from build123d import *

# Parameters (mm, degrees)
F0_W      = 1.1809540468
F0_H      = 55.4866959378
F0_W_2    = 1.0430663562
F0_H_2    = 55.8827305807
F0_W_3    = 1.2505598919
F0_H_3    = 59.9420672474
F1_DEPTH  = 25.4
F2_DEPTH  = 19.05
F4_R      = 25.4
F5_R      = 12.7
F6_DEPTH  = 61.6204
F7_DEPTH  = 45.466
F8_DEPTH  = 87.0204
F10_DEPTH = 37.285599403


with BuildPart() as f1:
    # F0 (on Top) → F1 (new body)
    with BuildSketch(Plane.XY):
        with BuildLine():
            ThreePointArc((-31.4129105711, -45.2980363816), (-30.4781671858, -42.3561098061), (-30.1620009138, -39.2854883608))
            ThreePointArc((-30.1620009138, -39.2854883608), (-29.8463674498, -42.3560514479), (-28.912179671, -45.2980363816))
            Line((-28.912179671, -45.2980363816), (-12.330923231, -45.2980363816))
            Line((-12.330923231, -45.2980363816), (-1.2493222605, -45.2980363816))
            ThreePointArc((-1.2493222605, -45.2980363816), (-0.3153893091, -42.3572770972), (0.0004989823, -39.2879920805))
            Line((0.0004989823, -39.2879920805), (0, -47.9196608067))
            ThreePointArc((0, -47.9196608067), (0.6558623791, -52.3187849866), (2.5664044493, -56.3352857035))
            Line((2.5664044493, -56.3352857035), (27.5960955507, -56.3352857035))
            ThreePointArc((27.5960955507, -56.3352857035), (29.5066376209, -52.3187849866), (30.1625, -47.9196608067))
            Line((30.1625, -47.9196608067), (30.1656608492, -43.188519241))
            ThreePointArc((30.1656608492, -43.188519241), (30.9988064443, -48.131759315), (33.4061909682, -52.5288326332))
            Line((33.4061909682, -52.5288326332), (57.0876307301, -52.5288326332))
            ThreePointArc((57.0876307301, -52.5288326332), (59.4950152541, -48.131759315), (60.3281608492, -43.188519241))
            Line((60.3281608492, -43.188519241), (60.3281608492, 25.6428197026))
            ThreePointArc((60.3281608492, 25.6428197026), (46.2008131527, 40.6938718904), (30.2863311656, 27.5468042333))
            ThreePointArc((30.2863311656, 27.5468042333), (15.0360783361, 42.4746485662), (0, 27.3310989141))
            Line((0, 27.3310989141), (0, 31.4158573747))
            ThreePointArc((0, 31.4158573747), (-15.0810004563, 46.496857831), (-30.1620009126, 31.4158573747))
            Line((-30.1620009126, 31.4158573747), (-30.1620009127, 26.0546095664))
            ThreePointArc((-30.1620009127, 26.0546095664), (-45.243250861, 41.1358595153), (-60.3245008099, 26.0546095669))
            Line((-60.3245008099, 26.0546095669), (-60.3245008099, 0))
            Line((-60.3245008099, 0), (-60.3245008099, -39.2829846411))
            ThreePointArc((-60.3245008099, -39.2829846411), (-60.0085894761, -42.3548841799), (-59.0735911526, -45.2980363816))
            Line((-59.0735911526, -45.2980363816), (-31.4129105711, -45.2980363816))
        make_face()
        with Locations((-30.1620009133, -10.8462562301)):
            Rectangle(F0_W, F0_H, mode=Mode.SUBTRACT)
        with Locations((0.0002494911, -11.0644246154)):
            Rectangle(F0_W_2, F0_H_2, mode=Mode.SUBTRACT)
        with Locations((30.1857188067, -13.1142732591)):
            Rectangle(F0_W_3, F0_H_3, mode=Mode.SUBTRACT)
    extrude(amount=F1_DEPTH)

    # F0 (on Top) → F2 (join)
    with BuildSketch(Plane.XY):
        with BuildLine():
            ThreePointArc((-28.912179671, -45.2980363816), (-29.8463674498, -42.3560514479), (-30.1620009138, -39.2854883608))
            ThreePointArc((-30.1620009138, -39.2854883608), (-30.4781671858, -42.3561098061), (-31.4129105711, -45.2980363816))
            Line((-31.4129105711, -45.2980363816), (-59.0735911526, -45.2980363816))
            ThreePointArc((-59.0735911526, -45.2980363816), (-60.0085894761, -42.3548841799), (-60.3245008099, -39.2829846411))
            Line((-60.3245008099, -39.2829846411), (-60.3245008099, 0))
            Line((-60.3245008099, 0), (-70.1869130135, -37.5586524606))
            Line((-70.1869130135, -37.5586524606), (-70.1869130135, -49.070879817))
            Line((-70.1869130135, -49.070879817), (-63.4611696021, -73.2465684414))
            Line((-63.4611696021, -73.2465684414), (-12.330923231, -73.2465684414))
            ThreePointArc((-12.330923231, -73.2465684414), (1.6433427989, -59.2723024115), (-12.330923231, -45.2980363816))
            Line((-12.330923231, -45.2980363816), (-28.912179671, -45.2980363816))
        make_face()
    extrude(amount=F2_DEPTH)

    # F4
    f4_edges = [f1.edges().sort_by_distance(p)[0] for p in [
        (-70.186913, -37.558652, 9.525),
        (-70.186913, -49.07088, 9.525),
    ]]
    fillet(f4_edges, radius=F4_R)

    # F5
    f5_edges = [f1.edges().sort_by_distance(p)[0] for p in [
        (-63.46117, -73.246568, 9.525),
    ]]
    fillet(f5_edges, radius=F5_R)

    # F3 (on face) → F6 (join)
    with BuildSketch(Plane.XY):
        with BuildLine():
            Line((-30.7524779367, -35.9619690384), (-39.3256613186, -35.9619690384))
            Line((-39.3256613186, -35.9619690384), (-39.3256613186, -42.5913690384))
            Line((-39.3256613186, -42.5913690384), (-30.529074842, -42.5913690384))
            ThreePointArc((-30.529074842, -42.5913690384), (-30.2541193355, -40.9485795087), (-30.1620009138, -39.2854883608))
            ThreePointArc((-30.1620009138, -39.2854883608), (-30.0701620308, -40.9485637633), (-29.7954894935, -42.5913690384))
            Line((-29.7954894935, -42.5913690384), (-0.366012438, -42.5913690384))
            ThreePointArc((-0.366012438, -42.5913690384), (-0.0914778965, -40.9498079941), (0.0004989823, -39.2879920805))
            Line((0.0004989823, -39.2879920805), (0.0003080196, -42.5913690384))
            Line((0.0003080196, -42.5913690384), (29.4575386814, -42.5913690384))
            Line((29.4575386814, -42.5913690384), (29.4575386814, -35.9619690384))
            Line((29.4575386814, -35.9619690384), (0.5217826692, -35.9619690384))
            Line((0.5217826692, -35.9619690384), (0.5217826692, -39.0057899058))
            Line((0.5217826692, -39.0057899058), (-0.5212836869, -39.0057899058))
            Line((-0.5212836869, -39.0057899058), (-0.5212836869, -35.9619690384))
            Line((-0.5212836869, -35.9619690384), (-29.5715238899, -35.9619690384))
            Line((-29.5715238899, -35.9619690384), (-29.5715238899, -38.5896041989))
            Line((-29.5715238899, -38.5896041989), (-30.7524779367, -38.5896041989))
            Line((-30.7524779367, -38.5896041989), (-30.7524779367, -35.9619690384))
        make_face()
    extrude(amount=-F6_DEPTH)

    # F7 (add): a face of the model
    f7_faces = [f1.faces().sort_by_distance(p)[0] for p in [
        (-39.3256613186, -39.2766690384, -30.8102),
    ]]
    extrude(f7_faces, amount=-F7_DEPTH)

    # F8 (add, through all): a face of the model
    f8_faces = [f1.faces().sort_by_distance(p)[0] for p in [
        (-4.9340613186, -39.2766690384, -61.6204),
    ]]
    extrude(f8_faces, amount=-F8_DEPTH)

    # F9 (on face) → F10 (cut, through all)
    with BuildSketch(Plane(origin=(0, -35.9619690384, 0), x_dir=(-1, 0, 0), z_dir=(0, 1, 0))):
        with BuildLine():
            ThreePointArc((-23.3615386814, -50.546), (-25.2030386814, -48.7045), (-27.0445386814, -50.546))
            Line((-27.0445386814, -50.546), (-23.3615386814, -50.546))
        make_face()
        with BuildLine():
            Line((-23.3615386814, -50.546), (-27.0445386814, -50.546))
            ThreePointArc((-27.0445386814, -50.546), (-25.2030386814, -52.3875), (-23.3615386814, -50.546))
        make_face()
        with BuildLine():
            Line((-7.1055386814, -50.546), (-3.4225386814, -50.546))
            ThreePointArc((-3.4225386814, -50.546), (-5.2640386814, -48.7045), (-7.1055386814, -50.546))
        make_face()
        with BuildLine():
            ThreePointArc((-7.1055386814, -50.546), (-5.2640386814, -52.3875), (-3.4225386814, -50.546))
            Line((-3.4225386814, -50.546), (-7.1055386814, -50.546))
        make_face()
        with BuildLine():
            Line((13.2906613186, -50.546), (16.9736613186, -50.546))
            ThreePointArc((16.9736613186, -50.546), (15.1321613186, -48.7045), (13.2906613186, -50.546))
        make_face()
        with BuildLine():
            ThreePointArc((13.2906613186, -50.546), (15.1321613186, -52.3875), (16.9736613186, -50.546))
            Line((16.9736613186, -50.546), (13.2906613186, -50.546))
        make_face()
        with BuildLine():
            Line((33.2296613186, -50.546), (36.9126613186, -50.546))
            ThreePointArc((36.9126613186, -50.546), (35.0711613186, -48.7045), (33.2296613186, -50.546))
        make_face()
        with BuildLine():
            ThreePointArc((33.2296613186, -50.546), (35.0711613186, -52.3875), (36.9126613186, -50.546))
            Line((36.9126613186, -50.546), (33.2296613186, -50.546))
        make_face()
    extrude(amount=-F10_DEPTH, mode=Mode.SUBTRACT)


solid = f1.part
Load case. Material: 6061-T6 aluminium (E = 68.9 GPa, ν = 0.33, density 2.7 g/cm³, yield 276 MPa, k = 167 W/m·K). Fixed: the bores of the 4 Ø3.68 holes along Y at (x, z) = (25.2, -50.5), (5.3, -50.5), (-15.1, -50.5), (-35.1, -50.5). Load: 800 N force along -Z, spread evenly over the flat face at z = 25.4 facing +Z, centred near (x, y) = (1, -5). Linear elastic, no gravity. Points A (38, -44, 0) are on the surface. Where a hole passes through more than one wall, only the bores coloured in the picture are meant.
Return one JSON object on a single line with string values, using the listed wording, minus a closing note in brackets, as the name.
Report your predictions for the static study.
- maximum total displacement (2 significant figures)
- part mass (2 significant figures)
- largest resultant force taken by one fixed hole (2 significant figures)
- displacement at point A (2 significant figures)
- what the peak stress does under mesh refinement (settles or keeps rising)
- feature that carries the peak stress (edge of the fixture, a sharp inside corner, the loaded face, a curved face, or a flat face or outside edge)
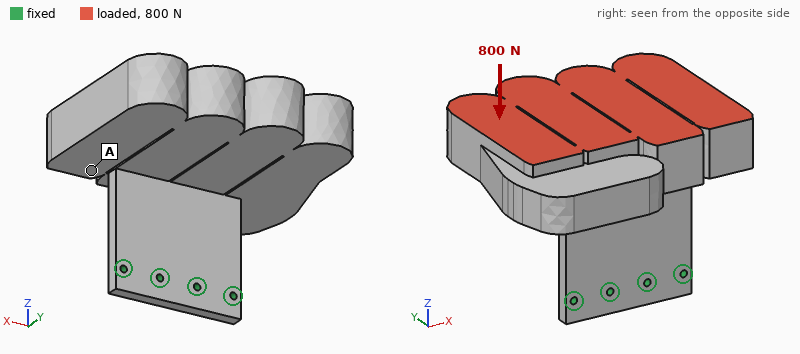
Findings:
{"maximum total displacement": "1.2 mm", "part mass": "910 g", "largest resultant force taken by one fixed hole": "280 N", "displacement at point A": "0.30 mm", "what the peak stress does under mesh refinement": "keeps rising", "feature that carries the peak stress": "edge of the fixture"}
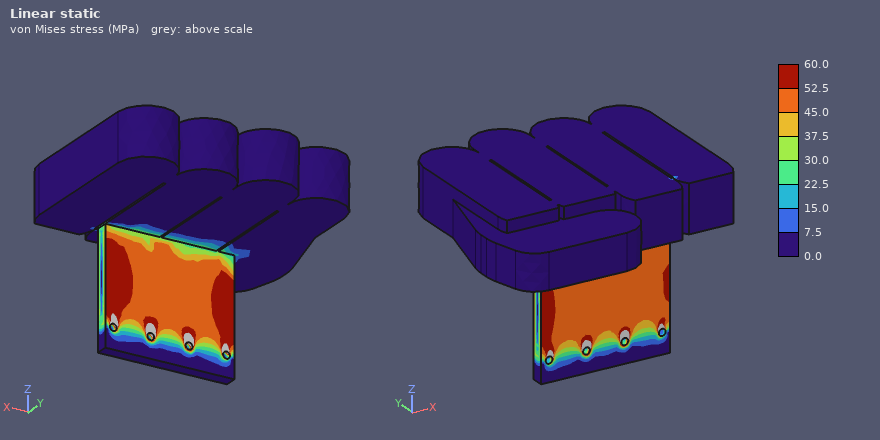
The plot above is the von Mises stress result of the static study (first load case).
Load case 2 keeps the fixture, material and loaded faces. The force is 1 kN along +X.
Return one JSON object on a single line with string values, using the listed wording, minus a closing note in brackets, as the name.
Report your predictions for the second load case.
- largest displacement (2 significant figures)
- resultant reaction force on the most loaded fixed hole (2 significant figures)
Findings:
{"largest displacement": "0.49 mm", "resultant reaction force on the most loaded fixed hole": "1.2 kN"}
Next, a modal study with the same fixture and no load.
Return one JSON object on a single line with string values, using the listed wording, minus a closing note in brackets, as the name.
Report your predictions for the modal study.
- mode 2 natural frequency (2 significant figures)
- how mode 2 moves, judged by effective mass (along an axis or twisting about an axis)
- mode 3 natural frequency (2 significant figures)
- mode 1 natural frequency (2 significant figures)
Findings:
{"mode 2 natural frequency": "270 Hz", "how mode 2 moves, judged by effective mass": "along X", "mode 3 natural frequency": "700 Hz", "mode 1 natural frequency": "150 Hz"}
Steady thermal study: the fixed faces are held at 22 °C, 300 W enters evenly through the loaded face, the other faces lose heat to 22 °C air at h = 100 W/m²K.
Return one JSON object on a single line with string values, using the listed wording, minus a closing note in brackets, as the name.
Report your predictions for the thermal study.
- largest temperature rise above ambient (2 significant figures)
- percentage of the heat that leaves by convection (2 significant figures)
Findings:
{"largest temperature rise above ambient": "69 K", "percentage of the heat that leaves by convection": "78 %"}
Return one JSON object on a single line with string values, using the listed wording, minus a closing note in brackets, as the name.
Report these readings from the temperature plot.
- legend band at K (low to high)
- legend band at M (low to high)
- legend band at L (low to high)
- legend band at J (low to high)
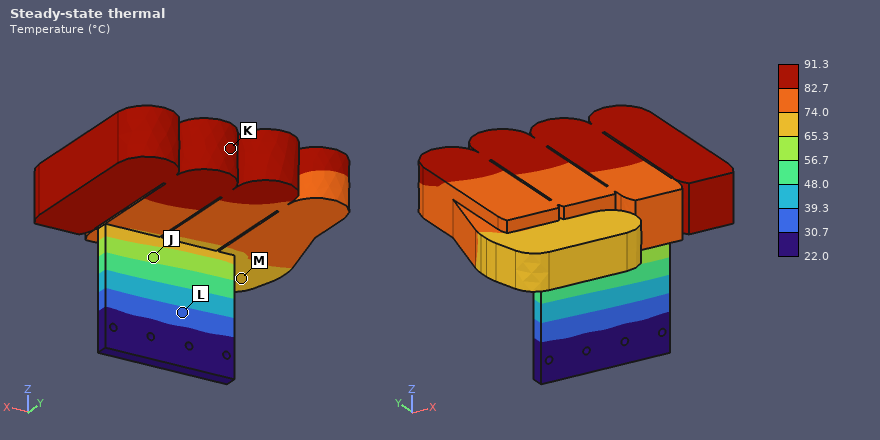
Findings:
{"legend band at K": "82.7 to 91.3 °C", "legend band at M": "65.3 to 74.0 °C", "legend band at L": "30.7 to 39.3 °C", "legend band at J": "56.7 to 65.3 °C"}
